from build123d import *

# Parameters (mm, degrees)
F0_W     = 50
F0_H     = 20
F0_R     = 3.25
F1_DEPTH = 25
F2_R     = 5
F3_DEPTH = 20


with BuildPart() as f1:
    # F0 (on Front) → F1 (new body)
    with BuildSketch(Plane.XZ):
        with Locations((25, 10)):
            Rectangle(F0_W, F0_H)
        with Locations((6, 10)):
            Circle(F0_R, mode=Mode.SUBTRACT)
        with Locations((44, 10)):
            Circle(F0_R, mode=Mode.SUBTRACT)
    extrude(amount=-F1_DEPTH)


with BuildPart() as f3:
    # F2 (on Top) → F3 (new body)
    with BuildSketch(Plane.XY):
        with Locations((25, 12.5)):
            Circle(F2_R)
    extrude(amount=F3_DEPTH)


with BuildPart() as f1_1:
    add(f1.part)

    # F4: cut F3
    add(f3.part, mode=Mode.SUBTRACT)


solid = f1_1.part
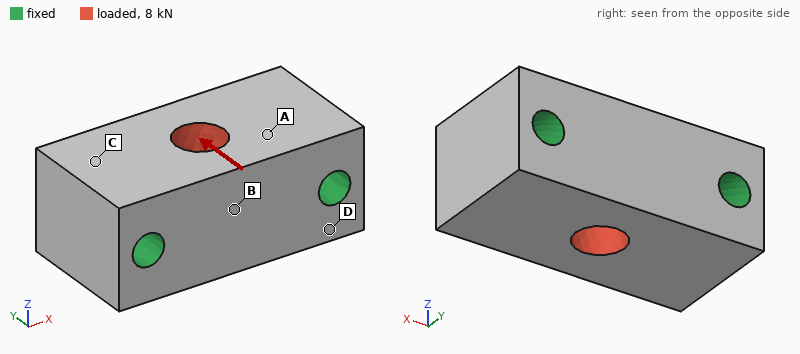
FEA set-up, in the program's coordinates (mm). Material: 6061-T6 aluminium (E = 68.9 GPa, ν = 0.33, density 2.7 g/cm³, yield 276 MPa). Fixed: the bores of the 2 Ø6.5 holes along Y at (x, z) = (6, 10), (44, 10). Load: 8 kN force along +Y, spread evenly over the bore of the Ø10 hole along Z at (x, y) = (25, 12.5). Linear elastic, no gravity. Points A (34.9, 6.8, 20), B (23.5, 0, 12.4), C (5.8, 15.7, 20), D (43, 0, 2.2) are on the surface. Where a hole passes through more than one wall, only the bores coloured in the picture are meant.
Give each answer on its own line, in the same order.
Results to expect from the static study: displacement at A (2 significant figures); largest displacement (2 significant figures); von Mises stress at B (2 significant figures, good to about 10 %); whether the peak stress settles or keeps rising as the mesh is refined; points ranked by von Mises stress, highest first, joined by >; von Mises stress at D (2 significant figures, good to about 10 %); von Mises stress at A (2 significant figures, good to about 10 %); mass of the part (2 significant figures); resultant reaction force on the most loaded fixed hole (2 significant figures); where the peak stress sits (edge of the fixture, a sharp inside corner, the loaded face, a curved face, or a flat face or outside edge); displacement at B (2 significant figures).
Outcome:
3.6 µm
7.5 µm
20 MPa
keeps rising
B > A > D > C
7.2 MPa
15 MPa
59 g
4.0 kN
edge of the fixture
6.1 µm
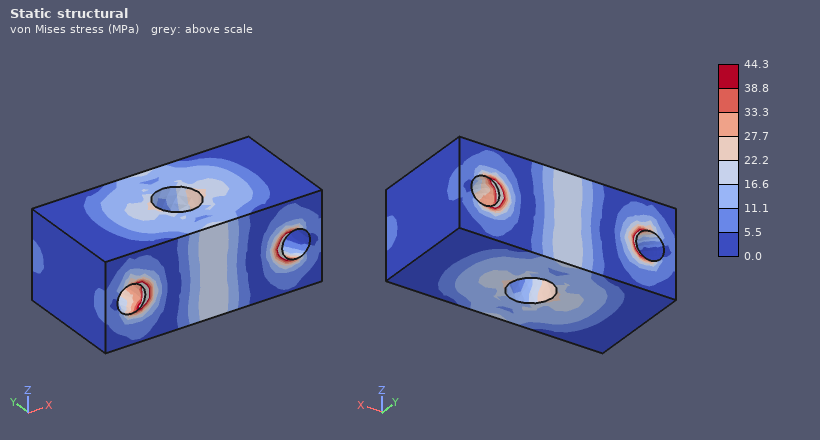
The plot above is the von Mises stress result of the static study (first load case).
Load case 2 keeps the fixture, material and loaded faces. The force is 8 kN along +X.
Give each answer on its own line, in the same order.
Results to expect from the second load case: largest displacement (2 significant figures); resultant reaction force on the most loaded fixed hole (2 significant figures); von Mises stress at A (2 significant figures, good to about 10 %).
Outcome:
2.8 µm
4.0 kN
7.9 MPa
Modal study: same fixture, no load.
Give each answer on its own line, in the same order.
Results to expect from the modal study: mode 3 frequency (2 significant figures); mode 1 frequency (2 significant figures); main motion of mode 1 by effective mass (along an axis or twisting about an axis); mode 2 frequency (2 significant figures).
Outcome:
39 kHz
32 kHz
along Z
39 kHz
